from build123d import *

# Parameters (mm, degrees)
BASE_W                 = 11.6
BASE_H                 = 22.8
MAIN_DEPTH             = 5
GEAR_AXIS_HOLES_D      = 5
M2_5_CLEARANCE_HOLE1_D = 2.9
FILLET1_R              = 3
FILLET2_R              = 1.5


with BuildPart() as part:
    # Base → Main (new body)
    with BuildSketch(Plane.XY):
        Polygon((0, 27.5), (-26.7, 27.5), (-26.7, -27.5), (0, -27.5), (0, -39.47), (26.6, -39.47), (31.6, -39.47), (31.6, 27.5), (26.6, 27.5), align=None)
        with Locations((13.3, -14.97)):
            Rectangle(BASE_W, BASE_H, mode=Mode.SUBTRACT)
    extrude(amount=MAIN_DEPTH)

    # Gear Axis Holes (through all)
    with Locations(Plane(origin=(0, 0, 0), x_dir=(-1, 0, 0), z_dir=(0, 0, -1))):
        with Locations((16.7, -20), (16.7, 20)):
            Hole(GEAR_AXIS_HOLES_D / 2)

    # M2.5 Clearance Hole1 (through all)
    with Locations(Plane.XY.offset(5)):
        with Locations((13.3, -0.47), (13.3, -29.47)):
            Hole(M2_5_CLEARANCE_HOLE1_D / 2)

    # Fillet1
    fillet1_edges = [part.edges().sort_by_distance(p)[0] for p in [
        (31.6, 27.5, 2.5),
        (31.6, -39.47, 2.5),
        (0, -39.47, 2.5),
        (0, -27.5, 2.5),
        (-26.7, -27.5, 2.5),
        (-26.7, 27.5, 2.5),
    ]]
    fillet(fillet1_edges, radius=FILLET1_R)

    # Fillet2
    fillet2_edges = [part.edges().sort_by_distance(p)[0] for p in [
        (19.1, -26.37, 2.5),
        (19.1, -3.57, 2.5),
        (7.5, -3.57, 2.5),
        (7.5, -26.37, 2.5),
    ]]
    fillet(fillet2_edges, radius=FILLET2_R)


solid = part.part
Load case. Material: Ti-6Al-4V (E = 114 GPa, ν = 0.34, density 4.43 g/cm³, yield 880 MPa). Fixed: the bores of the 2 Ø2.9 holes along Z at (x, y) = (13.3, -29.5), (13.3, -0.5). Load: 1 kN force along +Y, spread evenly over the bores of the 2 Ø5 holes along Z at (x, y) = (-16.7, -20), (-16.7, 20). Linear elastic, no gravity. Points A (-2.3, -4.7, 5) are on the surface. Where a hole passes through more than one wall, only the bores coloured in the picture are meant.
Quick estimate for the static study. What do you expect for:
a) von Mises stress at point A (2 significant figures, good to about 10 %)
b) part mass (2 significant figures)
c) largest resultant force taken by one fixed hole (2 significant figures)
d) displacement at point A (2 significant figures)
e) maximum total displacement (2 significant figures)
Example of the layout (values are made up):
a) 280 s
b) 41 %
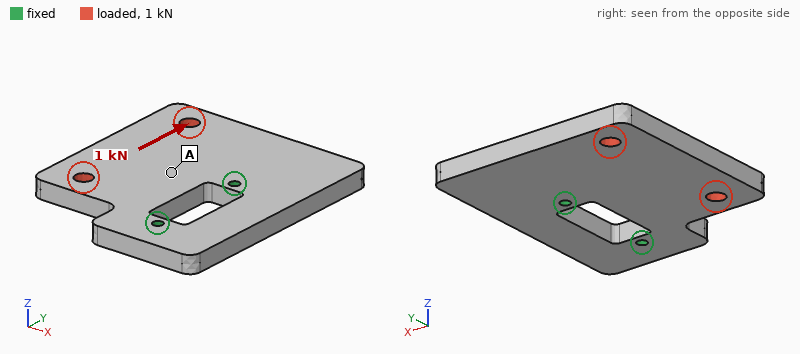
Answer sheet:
a) 11 MPa
b) 72 g
c) 1.1 kN
d) 5.9 µm
e) 16 µm
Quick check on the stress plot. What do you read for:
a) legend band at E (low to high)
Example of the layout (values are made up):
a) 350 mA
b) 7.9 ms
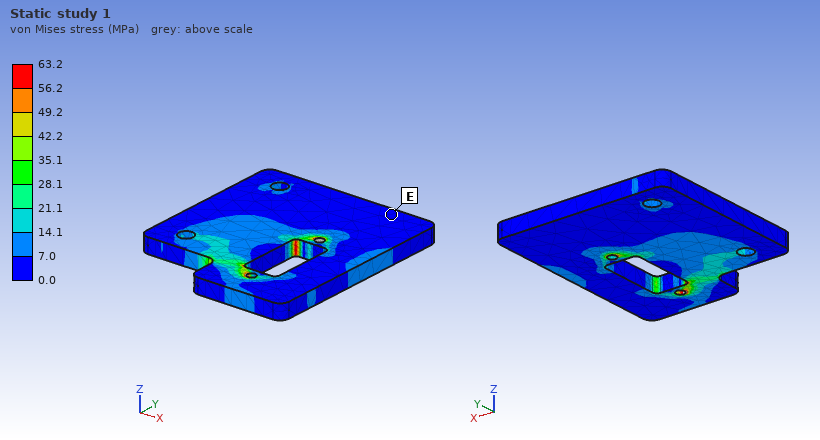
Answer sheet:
a) 0.0 to 7.0 MPa
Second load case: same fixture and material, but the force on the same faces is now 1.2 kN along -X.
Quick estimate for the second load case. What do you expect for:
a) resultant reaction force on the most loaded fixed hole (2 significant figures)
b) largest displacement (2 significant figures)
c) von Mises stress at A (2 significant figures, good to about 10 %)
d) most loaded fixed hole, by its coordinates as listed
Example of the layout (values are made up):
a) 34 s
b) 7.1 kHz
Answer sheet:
a) 1.2 kN
b) 8.3 µm
c) 8.5 MPa
d) (13.3, -0.5)
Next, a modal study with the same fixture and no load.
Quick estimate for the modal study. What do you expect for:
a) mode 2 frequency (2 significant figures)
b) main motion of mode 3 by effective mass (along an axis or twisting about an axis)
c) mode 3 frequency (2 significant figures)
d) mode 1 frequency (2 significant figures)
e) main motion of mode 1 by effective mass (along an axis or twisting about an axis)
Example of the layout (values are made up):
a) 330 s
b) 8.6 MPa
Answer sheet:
a) 3500 Hz
b) along Z
c) 5400 Hz
d) 1800 Hz
e) along Z
